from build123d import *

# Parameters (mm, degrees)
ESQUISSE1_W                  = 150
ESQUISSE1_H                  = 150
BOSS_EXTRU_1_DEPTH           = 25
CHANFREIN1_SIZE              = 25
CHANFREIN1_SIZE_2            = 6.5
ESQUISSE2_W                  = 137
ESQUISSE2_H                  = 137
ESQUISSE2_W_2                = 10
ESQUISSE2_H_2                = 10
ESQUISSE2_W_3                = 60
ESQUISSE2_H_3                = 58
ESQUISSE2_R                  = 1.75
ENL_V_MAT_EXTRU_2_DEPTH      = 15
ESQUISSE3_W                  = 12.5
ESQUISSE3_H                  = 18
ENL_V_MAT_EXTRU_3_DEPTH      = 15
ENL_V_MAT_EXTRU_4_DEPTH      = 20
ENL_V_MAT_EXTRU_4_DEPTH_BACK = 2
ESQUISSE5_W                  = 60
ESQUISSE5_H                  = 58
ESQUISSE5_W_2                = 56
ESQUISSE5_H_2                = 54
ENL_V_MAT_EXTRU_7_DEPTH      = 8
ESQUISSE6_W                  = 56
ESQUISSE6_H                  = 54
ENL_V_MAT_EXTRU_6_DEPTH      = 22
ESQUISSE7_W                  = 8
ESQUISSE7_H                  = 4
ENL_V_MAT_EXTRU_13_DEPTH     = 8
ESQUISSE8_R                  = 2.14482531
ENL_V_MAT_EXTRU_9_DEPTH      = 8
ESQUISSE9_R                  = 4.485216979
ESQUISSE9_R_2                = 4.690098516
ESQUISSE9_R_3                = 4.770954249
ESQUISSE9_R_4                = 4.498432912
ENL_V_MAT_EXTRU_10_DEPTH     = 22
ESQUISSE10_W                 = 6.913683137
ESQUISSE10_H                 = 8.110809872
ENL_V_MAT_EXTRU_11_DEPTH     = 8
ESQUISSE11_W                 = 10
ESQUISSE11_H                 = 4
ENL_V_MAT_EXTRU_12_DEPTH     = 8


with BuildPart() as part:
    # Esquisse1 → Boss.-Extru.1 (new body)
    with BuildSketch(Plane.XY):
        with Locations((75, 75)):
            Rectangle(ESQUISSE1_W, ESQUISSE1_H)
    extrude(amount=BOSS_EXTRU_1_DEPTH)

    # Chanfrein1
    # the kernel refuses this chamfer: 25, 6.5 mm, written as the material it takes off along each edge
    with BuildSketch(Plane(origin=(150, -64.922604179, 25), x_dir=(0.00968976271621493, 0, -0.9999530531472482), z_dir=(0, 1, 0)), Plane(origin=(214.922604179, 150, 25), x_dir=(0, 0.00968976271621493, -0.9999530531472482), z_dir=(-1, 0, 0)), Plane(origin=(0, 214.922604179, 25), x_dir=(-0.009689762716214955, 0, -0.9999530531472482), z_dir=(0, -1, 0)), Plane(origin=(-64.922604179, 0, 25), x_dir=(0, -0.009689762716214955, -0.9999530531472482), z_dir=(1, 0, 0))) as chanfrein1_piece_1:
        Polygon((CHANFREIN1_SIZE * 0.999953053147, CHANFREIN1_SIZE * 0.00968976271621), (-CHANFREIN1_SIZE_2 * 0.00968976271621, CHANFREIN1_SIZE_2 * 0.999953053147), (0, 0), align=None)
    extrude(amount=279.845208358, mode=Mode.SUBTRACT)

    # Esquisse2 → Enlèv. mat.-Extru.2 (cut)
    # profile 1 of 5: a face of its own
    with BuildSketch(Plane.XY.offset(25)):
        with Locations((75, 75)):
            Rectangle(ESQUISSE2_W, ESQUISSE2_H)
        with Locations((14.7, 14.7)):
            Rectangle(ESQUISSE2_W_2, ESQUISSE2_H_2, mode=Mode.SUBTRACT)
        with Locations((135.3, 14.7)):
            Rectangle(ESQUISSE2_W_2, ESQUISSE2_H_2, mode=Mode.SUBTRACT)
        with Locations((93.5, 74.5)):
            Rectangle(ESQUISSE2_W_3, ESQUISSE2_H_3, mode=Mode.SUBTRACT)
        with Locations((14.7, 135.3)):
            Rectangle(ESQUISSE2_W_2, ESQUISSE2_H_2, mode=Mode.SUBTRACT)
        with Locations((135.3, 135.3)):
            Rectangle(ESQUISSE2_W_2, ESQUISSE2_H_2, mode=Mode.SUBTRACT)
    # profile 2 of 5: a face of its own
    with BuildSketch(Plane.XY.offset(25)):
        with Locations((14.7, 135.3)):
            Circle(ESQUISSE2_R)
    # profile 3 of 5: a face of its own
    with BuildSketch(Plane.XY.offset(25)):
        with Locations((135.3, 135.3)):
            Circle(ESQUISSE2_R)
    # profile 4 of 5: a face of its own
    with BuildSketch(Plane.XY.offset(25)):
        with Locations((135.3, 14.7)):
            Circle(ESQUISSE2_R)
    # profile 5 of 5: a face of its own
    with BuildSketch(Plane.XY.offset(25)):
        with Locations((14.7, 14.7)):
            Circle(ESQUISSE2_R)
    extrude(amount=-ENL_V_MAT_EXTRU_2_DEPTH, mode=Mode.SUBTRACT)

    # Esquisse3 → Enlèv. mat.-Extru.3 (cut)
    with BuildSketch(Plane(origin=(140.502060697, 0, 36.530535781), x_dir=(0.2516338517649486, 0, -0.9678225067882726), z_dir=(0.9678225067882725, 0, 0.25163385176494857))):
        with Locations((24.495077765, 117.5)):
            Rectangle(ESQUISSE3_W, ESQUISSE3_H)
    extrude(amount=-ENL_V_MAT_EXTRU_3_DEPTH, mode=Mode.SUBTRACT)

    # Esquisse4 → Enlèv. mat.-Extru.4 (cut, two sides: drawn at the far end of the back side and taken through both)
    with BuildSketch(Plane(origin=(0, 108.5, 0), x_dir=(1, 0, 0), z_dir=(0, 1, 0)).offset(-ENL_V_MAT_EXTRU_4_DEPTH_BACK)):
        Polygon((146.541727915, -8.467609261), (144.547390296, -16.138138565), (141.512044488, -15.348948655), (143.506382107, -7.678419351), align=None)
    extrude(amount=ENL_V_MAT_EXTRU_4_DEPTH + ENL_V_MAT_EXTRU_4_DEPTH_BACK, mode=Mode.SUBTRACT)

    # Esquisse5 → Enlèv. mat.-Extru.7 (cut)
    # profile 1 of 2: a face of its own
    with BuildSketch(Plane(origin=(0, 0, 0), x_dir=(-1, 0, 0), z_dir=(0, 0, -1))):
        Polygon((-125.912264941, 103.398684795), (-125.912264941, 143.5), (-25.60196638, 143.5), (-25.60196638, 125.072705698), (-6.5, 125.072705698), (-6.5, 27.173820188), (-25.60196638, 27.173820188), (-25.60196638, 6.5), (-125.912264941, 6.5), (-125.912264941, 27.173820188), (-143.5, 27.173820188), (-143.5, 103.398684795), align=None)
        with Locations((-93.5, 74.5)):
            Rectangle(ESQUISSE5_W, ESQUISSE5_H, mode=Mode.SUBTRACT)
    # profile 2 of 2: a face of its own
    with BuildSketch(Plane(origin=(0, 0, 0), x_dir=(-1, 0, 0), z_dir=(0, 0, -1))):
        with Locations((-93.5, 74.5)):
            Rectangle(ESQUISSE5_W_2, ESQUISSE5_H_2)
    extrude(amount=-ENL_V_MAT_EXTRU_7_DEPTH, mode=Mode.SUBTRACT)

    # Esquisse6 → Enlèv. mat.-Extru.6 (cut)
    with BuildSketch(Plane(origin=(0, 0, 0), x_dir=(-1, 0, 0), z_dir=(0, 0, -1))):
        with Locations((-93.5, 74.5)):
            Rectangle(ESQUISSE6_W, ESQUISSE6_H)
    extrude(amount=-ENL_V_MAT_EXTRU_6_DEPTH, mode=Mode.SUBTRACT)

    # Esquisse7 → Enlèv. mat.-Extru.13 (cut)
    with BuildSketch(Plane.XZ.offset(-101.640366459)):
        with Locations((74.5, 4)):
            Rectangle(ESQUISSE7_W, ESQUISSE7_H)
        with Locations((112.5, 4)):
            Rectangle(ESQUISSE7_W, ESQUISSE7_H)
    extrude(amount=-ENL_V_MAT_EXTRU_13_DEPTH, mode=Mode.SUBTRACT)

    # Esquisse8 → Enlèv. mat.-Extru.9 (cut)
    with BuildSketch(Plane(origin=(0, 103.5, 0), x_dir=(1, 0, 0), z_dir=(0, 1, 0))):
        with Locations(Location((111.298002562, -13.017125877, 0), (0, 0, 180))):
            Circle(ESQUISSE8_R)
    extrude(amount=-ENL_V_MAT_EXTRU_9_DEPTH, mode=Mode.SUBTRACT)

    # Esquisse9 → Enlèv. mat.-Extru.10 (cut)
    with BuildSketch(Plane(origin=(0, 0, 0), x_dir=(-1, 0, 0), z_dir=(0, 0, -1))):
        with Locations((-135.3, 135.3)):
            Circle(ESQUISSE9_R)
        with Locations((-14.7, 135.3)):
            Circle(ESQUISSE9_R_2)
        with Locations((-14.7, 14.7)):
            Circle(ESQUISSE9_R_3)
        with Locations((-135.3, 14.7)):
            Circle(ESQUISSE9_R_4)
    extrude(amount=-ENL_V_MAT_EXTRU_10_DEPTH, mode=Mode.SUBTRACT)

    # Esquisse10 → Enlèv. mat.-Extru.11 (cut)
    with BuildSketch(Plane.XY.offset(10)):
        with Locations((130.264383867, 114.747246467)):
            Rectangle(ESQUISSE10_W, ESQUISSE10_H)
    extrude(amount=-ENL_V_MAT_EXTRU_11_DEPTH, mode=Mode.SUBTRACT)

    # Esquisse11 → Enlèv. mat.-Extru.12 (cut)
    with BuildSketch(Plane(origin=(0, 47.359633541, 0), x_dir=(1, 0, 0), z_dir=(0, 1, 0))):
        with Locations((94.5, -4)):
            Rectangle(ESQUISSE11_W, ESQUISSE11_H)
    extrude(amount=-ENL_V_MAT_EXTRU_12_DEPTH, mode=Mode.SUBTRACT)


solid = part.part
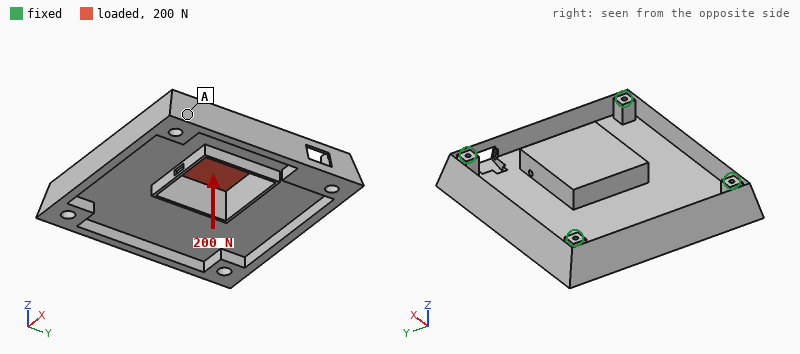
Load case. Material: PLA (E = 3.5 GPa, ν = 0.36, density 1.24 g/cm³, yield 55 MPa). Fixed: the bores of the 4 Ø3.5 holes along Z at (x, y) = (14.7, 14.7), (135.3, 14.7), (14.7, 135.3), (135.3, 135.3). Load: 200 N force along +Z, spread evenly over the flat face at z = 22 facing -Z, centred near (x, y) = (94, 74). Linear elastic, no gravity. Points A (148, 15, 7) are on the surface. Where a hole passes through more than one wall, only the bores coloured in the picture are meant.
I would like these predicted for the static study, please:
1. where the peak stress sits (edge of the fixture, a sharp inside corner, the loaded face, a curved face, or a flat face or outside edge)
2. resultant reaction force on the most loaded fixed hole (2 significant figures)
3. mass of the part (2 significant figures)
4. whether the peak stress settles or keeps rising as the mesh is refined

a sharp inside corner
83 N
140 g
keeps rising
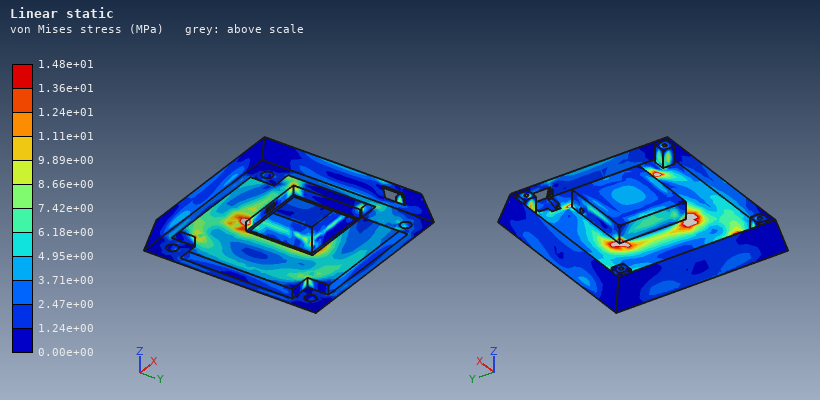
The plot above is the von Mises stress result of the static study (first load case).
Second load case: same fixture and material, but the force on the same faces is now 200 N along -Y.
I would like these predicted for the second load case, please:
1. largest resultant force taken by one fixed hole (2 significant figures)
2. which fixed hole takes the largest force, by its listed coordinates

67 N
(135.3, 14.7)
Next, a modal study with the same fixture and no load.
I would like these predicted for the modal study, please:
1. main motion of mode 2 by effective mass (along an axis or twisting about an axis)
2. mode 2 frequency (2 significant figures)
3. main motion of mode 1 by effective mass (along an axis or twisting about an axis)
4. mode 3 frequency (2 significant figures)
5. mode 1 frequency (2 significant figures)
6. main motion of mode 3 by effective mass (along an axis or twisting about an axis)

along Y
590 Hz
along Z
650 Hz
300 Hz
along X
